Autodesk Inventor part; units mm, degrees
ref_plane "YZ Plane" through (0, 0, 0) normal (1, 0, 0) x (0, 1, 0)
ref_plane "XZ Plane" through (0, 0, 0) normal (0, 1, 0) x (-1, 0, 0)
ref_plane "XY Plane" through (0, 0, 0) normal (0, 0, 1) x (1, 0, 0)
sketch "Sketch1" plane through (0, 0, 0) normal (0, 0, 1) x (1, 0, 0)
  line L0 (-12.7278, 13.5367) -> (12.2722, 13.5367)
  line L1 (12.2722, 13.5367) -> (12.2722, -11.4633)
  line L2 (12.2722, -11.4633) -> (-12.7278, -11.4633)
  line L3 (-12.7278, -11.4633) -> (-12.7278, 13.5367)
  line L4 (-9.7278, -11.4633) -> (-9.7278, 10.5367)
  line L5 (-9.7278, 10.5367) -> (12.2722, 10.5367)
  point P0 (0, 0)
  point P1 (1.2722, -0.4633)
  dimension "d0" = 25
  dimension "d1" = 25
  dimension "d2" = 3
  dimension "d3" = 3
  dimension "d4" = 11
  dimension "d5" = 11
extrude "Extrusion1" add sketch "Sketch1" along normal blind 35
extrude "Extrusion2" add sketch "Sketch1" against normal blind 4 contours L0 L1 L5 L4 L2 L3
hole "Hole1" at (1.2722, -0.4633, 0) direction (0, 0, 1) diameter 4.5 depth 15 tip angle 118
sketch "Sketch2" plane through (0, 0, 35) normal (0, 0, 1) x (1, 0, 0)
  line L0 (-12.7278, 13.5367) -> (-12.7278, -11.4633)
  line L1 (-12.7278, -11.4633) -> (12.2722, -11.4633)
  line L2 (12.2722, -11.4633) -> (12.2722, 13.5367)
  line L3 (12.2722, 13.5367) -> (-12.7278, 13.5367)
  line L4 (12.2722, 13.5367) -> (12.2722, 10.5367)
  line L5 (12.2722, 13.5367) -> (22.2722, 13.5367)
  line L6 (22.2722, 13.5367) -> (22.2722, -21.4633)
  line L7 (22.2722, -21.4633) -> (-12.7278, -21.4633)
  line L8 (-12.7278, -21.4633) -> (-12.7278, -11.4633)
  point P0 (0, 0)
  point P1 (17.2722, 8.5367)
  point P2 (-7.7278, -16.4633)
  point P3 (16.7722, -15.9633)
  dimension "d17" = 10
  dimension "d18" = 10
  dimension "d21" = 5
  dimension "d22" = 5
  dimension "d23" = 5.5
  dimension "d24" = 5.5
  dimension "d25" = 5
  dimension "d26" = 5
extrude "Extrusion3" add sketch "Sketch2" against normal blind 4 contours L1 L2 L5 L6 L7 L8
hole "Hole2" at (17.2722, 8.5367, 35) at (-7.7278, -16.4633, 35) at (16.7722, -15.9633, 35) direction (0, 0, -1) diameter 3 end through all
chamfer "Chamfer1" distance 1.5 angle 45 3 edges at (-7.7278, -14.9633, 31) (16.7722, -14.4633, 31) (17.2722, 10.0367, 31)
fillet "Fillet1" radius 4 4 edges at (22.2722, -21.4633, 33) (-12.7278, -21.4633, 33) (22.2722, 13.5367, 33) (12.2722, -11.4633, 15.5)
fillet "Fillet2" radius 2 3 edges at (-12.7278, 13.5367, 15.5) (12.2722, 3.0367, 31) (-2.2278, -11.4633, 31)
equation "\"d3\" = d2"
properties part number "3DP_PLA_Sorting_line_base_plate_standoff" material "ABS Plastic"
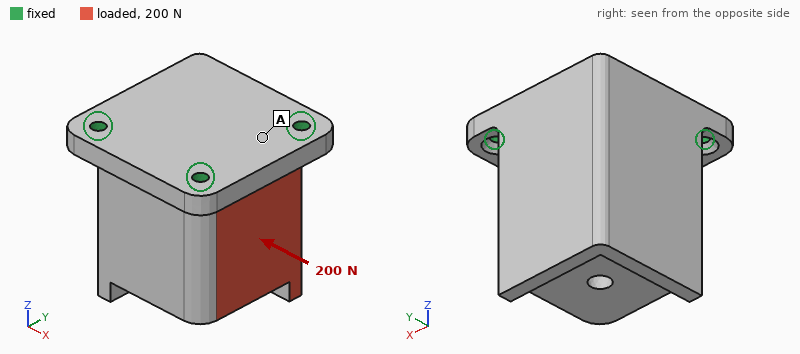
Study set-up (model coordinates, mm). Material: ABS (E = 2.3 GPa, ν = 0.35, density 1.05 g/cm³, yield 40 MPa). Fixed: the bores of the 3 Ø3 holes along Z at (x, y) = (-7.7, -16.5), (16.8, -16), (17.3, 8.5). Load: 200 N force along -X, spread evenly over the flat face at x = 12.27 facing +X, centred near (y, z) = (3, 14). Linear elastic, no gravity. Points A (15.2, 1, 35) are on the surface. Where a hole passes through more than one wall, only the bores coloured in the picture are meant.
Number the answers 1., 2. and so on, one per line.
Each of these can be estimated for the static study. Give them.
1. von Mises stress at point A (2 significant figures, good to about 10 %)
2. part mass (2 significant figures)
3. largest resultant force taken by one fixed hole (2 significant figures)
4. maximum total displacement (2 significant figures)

1. 3.7 MPa
2. 26 g
3. 200 N
4. 0.52 mm
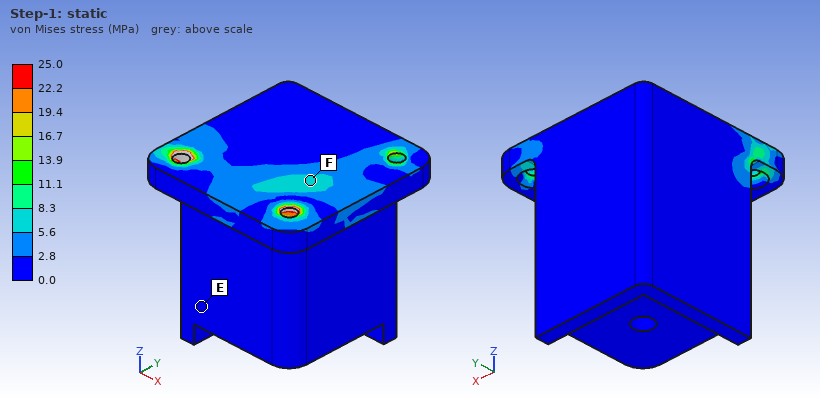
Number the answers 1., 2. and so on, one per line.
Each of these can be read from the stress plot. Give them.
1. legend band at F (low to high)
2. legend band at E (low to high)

1. 5.6 to 8.3 MPa
2. 0.0 to 2.8 MPa
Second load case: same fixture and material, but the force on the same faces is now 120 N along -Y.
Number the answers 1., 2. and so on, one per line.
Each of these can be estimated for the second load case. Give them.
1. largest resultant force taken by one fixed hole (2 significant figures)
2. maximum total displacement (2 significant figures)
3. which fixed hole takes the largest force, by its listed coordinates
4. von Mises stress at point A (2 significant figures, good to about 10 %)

1. 120 N
2. 0.31 mm
3. (16.8, -16)
4. 1.6 MPa
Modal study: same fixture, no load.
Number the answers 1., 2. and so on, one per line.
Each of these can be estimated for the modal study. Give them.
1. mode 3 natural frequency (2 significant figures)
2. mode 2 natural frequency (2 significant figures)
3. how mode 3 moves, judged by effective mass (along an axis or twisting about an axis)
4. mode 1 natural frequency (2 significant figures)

1. 2700 Hz
2. 1800 Hz
3. along Z
4. 710 Hz
